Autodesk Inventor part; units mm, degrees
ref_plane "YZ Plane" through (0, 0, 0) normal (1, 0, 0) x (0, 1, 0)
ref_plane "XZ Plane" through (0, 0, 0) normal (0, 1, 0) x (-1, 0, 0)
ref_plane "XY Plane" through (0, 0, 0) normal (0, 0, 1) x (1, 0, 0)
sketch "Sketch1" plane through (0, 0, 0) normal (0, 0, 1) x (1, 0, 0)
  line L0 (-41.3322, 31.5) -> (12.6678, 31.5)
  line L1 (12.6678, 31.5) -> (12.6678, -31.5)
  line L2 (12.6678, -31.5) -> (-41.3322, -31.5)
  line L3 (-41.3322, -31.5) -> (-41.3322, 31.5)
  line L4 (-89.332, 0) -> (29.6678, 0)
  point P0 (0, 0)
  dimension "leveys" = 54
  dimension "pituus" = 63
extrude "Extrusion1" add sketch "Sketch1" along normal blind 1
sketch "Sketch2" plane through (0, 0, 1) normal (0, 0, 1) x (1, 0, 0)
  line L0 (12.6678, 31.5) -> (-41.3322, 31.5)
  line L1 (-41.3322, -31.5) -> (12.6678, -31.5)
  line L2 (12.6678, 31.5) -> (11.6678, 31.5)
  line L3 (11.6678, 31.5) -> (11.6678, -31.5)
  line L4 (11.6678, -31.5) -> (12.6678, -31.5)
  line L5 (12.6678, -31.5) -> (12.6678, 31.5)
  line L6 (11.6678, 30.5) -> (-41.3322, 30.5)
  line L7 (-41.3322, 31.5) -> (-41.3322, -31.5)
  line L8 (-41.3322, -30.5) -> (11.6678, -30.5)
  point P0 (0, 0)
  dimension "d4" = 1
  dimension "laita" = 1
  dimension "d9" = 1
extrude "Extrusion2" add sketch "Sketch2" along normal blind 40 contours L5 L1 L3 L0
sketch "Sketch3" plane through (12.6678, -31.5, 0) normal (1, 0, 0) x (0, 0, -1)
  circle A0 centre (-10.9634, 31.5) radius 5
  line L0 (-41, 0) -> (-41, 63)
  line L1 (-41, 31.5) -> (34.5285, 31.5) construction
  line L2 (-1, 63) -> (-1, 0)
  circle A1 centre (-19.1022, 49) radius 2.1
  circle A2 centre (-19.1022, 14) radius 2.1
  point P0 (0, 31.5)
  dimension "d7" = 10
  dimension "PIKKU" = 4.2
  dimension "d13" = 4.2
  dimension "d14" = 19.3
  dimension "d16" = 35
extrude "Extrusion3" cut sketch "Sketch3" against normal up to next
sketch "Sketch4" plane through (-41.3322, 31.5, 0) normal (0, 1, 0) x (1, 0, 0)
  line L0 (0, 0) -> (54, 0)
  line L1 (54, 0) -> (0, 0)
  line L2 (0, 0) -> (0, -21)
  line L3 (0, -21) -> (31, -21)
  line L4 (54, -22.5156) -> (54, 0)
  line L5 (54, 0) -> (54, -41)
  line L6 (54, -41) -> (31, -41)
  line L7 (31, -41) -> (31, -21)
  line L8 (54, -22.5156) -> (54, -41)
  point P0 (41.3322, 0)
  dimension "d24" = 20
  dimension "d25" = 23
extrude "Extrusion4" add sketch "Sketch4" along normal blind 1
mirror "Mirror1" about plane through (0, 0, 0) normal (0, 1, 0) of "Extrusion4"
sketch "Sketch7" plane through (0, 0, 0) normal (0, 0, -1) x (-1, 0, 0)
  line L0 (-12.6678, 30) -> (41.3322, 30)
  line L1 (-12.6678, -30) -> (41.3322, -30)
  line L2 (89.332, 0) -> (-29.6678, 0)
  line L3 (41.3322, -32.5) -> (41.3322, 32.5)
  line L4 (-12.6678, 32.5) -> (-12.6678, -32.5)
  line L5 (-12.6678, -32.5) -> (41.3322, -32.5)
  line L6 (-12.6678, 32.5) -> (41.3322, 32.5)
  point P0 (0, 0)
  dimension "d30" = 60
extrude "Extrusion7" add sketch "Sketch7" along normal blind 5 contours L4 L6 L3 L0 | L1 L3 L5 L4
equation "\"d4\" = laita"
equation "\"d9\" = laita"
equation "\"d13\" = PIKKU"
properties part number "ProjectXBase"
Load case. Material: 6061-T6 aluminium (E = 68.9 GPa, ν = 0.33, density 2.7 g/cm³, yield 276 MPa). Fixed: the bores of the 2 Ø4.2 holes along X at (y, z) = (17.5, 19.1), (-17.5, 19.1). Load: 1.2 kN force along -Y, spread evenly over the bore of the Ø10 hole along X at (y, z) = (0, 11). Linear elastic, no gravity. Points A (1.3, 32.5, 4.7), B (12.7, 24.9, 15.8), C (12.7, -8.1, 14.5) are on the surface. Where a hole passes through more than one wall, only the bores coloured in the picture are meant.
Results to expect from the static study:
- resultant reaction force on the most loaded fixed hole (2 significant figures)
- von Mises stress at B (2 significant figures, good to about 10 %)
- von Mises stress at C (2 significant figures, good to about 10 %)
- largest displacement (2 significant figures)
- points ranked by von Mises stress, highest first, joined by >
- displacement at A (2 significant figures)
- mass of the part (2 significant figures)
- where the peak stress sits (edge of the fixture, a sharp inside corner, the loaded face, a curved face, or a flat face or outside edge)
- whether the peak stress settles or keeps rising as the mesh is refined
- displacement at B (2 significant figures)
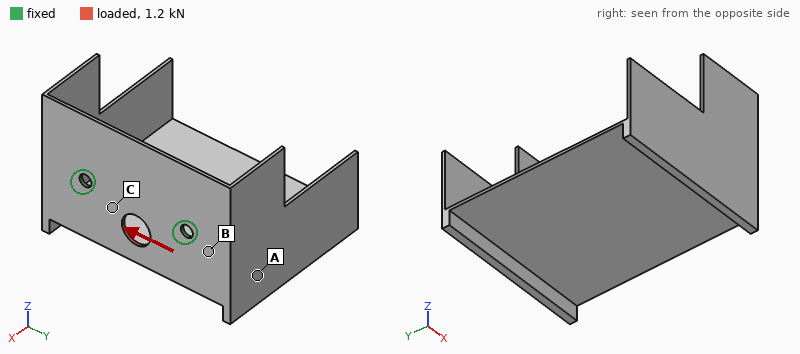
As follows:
650 N
15 MPa
45 MPa
19 µm
C > B > A
14 µm
28 g
edge of the fixture
keeps rising
5.2 µm
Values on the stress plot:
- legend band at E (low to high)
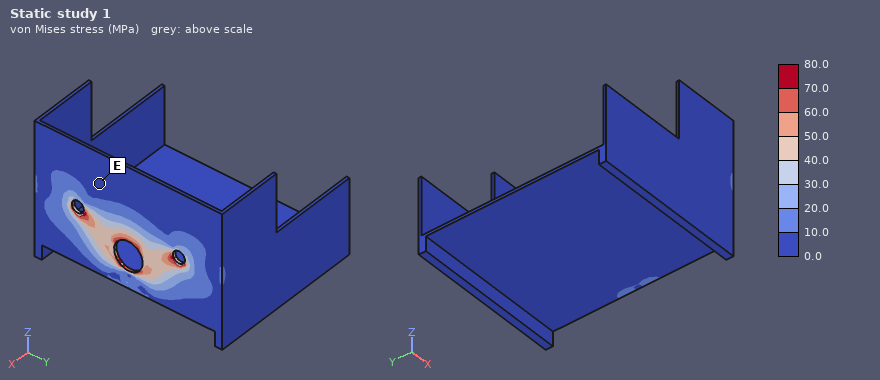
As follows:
0.0 to 10.0 MPa
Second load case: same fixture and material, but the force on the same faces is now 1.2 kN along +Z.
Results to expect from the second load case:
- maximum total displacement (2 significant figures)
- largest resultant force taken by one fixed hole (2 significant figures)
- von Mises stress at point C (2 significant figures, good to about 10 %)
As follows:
20 µm
610 N
39 MPa
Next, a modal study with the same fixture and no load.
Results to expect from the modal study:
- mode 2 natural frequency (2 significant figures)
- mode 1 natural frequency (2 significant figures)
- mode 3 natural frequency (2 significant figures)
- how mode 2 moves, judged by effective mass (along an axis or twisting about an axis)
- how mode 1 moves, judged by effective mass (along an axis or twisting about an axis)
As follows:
360 Hz
280 Hz
840 Hz
along Y
along Z
